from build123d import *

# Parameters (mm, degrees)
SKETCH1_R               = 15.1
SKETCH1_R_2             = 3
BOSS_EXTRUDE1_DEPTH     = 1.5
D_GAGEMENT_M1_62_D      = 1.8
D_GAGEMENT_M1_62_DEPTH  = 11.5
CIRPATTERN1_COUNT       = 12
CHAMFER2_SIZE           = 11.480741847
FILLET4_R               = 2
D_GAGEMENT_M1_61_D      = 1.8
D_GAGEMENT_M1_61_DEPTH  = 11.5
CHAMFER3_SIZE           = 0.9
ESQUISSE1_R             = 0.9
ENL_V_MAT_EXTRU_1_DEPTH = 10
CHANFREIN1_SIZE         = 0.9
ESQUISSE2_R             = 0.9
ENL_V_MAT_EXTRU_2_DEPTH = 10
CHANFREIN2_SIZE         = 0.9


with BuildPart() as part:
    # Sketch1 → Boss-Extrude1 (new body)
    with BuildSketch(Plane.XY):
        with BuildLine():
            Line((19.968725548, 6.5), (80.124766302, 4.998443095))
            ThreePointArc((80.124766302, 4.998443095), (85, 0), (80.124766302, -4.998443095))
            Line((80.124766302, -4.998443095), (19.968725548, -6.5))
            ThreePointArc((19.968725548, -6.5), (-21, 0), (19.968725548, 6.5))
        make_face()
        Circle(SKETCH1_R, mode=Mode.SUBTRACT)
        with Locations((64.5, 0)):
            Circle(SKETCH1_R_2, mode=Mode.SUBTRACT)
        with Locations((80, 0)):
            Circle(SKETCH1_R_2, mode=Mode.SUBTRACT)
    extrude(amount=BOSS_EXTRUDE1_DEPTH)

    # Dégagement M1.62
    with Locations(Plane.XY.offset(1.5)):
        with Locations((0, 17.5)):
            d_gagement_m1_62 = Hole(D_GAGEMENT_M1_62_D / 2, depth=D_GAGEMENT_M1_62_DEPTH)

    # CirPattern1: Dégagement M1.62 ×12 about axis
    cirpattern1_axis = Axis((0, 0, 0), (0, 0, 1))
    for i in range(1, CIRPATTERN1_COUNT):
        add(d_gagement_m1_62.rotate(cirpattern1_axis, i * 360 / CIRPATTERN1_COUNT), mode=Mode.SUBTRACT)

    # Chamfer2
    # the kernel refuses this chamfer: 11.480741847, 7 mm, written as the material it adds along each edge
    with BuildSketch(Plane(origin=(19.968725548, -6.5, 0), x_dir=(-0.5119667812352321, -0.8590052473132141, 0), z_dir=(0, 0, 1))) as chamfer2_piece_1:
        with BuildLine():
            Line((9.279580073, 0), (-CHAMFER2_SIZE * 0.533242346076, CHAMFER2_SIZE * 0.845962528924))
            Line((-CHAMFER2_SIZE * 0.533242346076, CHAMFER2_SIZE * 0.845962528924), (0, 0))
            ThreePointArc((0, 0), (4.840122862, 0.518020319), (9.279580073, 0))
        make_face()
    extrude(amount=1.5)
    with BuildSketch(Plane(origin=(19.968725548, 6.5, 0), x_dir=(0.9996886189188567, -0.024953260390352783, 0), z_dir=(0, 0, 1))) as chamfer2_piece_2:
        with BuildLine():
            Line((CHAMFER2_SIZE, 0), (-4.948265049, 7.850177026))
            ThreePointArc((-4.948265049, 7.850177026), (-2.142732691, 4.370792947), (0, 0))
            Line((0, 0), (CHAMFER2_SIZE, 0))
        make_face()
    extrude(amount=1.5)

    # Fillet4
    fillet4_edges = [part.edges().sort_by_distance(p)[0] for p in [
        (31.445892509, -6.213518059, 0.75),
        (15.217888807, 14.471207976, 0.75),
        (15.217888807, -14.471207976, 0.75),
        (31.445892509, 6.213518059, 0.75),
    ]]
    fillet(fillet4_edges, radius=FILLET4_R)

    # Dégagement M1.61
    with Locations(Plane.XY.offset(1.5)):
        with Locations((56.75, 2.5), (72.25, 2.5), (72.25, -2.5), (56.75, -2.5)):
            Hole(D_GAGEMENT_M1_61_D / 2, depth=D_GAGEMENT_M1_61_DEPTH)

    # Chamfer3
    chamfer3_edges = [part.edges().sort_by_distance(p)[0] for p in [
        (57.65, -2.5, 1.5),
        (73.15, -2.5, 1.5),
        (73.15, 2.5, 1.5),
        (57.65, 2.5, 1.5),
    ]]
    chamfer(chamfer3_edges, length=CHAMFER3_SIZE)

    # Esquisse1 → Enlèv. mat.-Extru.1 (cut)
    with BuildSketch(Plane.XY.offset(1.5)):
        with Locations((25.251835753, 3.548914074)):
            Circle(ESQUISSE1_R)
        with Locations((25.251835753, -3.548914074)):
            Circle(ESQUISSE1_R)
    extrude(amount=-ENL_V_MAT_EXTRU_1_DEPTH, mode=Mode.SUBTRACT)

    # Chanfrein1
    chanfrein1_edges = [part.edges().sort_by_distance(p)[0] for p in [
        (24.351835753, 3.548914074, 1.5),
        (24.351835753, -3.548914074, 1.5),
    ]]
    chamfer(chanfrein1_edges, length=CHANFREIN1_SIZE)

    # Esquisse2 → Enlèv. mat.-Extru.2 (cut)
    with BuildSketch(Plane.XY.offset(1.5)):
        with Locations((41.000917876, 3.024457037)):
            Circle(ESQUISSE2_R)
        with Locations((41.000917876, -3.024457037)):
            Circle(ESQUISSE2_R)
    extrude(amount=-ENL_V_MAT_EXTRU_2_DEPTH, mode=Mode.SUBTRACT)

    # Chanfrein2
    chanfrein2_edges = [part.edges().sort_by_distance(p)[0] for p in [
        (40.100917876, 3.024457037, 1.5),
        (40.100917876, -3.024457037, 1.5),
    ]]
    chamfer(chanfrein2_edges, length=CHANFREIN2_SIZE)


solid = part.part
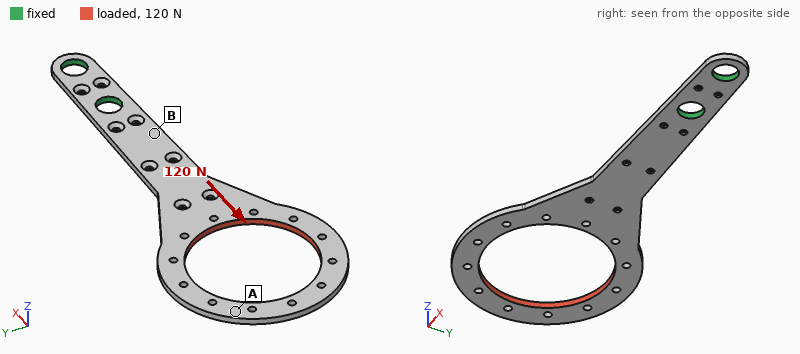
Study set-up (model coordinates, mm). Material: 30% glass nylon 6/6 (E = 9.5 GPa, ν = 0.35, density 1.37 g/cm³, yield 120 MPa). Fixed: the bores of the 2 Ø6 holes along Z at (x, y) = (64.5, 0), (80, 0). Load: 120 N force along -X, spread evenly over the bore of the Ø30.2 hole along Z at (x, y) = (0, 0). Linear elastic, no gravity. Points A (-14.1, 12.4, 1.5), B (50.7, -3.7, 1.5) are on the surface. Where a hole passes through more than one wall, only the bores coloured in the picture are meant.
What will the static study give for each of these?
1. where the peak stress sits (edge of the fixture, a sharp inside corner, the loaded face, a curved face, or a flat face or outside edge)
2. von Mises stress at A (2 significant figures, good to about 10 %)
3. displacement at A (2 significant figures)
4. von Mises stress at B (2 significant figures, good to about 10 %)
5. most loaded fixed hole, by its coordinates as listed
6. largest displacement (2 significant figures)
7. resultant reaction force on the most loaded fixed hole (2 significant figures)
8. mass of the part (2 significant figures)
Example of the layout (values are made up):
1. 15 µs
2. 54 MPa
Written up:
1. a curved face
2. 3.4 MPa
3. 0.28 mm
4. 6.9 MPa
5. (64.5, 0)
6. 0.32 mm
7. 120 N
8. 2.8 g
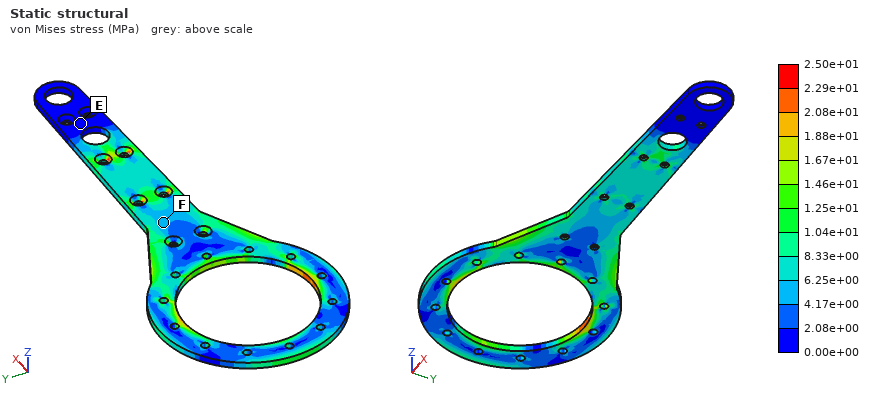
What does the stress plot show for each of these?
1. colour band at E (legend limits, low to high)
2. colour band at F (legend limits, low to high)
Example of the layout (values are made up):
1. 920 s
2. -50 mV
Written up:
1. 0.00e+00 to 2.08e+00 MPa
2. 4.17e+00 to 6.25e+00 MPa
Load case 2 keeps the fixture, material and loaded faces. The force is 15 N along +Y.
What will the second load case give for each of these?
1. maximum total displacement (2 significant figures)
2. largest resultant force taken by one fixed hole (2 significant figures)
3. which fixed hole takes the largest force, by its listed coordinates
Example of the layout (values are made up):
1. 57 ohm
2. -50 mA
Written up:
1. 1.2 mm
2. 22 N
3. (64.5, 0)
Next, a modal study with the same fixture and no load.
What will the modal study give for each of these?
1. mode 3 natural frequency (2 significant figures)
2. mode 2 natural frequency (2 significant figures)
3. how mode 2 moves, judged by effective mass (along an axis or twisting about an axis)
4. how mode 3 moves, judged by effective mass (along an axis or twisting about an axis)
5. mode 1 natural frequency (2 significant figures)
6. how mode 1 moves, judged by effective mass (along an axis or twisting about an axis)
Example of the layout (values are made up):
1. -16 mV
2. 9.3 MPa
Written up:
1. 470 Hz
2. 300 Hz
3. twisting about X
4. along Z
5. 75 Hz
6. along Z
